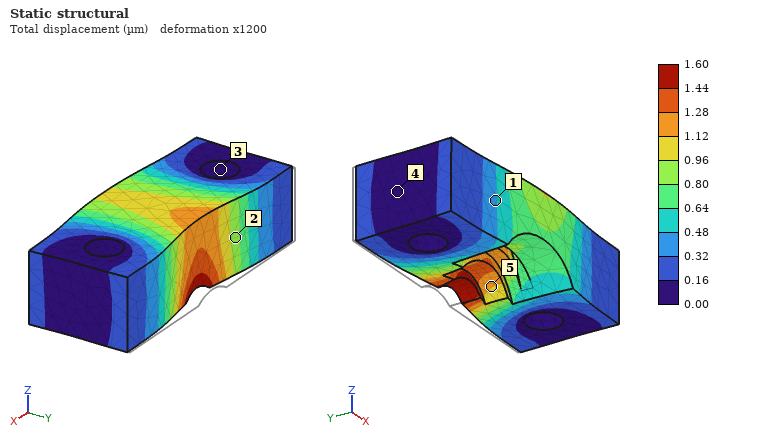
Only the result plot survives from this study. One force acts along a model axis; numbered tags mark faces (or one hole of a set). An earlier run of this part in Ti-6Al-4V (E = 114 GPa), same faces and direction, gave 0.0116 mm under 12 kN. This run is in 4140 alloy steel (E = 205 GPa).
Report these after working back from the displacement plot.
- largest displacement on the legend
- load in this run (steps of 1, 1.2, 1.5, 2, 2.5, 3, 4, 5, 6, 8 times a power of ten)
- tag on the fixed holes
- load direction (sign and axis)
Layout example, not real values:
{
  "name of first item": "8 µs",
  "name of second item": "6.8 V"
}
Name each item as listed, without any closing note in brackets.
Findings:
{
  "largest displacement on the legend": "1.60 µm",
  "load in this run": "3 kN",
  "tag on the fixed holes": "3",
  "load direction": "-Y"
}
